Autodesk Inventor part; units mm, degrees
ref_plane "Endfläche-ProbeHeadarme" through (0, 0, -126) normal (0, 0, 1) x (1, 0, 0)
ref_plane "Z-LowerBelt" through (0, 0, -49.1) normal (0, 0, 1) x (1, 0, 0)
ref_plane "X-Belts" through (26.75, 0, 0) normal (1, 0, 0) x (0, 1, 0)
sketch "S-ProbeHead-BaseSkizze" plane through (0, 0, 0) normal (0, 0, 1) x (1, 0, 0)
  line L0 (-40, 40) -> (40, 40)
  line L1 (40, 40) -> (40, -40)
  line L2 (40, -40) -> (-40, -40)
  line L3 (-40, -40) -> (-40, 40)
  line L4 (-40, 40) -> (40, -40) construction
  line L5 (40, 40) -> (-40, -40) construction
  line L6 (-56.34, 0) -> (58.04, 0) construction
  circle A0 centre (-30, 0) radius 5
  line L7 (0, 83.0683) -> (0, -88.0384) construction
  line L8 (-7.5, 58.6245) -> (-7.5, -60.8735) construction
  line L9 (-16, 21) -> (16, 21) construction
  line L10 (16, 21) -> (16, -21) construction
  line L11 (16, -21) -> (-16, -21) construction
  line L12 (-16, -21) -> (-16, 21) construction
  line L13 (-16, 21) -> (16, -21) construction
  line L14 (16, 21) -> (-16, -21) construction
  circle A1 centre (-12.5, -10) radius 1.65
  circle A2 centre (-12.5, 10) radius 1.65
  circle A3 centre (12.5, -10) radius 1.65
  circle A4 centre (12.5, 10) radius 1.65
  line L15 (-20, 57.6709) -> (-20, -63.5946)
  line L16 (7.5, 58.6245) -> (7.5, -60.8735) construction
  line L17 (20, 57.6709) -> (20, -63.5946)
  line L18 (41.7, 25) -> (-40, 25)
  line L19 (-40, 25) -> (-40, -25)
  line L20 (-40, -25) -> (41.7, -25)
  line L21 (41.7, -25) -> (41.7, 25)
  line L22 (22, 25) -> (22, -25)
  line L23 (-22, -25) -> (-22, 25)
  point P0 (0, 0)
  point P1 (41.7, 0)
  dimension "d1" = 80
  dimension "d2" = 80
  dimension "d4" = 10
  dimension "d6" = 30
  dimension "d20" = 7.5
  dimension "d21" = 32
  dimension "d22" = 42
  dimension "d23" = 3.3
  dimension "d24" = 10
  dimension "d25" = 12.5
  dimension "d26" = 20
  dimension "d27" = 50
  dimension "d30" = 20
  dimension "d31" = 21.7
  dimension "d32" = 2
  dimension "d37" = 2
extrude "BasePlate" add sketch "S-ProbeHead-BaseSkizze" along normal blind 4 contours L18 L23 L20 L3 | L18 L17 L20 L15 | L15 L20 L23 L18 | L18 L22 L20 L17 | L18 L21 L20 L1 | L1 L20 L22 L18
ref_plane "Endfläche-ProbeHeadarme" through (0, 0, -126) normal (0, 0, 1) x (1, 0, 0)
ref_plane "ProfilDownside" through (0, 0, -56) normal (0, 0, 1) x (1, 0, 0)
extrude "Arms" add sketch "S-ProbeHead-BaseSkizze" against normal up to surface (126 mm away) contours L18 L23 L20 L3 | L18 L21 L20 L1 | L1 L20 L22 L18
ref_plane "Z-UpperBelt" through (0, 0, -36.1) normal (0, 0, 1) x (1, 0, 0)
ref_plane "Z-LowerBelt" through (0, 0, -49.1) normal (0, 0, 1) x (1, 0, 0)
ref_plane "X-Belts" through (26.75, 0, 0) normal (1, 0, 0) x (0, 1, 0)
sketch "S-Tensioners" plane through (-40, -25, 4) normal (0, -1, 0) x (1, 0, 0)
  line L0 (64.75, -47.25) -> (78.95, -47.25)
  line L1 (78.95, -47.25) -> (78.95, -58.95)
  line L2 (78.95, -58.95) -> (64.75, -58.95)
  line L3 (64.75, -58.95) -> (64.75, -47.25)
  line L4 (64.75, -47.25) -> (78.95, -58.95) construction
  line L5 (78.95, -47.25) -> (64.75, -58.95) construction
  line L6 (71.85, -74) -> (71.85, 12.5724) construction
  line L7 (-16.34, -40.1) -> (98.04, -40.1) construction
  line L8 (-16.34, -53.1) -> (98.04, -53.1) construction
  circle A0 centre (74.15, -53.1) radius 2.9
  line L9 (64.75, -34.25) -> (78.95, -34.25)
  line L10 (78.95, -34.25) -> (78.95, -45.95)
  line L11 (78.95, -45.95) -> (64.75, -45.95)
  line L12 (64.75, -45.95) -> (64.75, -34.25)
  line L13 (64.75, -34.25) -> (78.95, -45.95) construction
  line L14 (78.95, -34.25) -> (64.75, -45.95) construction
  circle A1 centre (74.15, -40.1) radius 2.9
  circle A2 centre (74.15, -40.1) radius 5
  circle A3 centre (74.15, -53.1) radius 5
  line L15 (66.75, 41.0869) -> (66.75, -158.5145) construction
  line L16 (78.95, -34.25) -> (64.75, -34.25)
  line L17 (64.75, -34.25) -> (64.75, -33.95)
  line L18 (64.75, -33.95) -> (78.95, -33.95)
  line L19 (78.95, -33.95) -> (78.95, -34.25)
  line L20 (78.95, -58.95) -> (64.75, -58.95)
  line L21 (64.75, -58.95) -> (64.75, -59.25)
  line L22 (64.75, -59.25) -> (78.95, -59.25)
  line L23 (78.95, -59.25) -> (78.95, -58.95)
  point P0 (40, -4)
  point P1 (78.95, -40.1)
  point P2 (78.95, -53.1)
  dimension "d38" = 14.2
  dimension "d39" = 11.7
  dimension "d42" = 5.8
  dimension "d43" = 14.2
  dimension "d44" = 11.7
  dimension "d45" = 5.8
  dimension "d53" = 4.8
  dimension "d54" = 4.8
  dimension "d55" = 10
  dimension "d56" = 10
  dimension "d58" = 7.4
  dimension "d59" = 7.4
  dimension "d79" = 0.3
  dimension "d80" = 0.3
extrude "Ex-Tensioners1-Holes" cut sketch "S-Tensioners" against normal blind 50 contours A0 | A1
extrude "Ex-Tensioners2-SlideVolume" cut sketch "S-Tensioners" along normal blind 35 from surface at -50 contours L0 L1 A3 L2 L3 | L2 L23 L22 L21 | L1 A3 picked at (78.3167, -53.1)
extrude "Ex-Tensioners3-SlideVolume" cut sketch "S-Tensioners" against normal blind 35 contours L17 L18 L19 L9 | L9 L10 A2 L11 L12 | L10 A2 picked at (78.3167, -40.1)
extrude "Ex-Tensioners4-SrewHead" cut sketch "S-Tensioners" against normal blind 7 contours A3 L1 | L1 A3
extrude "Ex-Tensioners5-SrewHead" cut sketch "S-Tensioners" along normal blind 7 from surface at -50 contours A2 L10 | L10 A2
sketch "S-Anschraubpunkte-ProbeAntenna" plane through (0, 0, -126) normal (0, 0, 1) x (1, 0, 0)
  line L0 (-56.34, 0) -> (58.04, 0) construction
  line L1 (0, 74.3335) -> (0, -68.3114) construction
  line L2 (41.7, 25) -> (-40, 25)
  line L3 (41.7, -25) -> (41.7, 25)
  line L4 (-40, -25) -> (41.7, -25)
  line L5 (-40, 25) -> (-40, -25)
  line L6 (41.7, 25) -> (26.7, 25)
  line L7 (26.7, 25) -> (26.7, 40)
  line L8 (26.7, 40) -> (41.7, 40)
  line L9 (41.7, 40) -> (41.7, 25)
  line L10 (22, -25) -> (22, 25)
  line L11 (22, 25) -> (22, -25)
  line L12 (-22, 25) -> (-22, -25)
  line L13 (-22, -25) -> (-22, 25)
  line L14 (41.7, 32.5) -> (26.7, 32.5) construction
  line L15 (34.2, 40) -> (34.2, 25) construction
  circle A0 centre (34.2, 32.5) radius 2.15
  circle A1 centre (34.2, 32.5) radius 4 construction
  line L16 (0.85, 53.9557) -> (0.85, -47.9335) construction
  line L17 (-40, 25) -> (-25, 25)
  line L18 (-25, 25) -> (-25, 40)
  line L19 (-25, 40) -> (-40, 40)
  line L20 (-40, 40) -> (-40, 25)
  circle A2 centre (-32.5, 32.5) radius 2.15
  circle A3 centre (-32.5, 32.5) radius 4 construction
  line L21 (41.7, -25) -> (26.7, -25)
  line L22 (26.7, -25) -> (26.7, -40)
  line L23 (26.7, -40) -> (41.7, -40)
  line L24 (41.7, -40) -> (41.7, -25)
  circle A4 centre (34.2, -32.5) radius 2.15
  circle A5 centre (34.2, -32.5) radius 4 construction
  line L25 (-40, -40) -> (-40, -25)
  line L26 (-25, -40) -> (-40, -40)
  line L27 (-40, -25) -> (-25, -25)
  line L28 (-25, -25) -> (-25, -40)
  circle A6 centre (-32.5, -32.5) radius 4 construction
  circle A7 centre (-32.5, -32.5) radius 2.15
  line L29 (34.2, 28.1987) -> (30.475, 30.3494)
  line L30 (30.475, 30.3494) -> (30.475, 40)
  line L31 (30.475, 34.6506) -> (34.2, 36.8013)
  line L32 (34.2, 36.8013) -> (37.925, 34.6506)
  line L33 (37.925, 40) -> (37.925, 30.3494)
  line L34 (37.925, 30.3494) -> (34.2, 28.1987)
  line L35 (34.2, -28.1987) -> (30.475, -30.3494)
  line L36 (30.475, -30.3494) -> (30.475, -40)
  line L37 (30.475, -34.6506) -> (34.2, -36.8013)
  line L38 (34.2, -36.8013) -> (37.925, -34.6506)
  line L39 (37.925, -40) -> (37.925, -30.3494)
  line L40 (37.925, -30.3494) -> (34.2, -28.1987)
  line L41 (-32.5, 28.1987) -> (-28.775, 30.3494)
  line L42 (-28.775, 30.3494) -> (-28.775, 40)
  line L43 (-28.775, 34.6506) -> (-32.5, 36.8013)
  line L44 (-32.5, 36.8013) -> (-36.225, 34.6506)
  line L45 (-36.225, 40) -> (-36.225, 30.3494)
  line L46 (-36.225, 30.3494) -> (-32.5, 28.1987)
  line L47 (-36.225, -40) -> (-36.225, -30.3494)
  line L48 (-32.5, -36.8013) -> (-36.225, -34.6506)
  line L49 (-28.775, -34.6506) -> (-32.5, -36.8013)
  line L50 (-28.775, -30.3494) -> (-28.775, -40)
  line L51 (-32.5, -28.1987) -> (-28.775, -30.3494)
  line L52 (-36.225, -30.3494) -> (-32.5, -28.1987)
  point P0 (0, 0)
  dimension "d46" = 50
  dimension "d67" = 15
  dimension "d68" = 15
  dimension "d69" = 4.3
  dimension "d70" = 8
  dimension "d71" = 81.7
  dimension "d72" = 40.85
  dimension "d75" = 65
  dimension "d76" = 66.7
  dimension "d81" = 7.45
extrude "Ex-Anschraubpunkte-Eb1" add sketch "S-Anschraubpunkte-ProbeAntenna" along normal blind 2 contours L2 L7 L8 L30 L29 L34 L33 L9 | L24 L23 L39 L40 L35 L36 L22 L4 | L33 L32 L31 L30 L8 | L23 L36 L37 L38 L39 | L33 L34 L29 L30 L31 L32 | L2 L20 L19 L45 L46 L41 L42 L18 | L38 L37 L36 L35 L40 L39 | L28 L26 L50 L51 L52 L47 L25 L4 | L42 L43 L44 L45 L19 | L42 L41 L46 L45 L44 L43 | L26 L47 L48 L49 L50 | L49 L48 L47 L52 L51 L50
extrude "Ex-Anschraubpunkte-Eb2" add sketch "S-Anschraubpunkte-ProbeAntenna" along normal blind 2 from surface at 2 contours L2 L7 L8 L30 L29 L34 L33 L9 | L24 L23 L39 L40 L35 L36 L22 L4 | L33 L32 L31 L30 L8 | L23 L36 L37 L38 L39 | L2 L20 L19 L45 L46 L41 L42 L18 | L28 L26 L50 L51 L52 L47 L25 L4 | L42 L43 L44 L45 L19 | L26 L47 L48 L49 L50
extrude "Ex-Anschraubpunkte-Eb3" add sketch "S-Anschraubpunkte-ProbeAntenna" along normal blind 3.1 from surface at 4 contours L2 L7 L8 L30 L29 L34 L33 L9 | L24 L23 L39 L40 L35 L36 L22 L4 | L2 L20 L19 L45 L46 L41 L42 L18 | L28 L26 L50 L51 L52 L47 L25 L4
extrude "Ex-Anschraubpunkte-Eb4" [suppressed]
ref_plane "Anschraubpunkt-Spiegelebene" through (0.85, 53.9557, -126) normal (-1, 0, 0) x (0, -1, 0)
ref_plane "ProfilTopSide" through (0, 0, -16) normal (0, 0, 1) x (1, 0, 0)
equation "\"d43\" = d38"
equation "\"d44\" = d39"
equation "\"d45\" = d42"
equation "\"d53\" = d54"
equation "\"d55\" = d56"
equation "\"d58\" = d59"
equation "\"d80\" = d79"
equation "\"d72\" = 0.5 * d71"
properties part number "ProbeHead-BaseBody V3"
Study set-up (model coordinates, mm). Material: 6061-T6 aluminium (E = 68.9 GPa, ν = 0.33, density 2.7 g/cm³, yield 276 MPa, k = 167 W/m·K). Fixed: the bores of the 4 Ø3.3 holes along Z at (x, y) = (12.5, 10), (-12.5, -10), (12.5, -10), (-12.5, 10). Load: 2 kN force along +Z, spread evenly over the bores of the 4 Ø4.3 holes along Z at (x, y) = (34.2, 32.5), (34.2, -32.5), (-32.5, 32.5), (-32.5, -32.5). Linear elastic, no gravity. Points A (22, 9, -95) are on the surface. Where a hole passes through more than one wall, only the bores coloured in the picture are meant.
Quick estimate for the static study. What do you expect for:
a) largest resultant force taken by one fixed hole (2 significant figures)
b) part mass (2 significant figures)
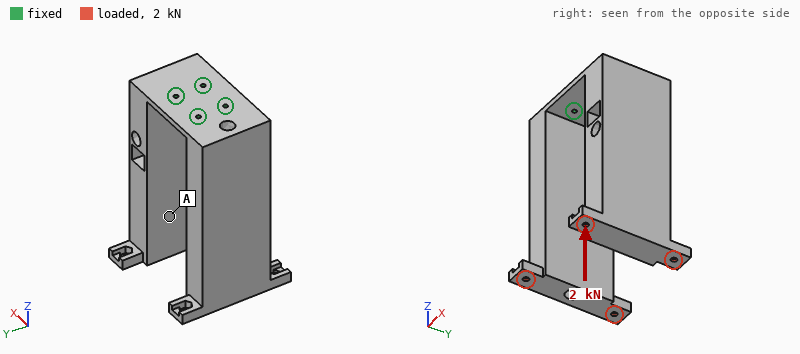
510 N
630 g
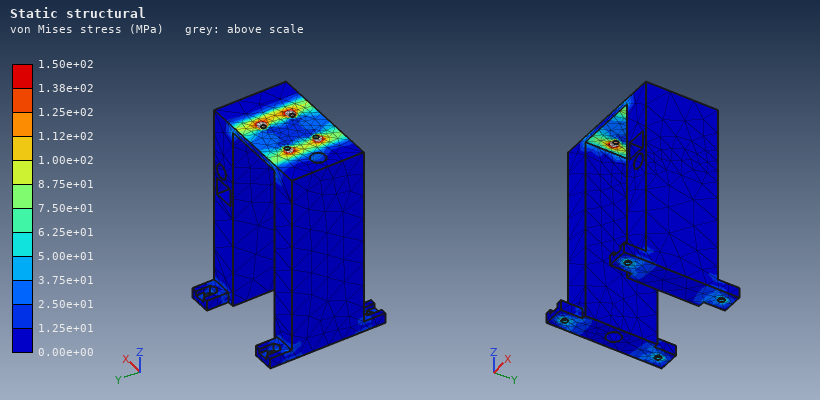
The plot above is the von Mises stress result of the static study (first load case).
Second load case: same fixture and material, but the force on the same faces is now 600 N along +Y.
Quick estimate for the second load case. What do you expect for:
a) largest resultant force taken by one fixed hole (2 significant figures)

1.5 kN
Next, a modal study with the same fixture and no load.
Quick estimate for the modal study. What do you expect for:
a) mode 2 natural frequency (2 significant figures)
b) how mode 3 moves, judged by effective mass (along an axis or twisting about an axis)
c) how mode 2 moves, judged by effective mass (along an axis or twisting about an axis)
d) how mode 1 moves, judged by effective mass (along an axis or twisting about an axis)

150 Hz
along Y
along X
along X
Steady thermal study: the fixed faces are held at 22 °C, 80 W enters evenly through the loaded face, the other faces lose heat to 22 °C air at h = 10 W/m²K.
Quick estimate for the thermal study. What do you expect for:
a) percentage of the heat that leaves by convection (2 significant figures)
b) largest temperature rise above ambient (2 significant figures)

22 %
76 K
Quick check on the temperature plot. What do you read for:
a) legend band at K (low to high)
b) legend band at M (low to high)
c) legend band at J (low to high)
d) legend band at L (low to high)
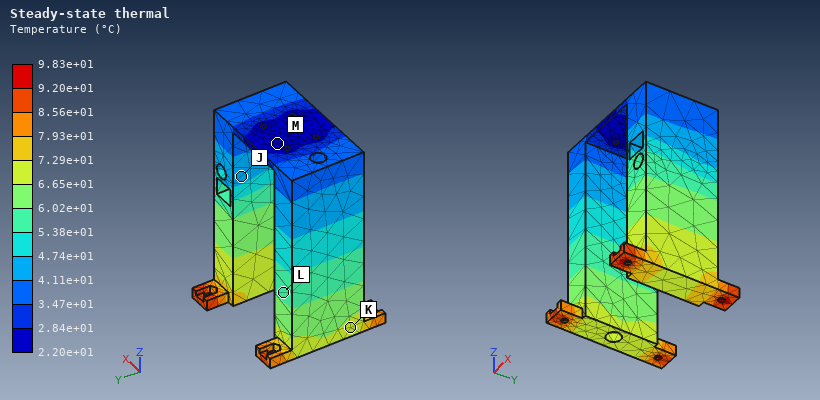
6.65e+01 to 7.29e+01 °C
2.20e+01 to 2.84e+01 °C
4.11e+01 to 4.74e+01 °C
5.38e+01 to 6.02e+01 °C
